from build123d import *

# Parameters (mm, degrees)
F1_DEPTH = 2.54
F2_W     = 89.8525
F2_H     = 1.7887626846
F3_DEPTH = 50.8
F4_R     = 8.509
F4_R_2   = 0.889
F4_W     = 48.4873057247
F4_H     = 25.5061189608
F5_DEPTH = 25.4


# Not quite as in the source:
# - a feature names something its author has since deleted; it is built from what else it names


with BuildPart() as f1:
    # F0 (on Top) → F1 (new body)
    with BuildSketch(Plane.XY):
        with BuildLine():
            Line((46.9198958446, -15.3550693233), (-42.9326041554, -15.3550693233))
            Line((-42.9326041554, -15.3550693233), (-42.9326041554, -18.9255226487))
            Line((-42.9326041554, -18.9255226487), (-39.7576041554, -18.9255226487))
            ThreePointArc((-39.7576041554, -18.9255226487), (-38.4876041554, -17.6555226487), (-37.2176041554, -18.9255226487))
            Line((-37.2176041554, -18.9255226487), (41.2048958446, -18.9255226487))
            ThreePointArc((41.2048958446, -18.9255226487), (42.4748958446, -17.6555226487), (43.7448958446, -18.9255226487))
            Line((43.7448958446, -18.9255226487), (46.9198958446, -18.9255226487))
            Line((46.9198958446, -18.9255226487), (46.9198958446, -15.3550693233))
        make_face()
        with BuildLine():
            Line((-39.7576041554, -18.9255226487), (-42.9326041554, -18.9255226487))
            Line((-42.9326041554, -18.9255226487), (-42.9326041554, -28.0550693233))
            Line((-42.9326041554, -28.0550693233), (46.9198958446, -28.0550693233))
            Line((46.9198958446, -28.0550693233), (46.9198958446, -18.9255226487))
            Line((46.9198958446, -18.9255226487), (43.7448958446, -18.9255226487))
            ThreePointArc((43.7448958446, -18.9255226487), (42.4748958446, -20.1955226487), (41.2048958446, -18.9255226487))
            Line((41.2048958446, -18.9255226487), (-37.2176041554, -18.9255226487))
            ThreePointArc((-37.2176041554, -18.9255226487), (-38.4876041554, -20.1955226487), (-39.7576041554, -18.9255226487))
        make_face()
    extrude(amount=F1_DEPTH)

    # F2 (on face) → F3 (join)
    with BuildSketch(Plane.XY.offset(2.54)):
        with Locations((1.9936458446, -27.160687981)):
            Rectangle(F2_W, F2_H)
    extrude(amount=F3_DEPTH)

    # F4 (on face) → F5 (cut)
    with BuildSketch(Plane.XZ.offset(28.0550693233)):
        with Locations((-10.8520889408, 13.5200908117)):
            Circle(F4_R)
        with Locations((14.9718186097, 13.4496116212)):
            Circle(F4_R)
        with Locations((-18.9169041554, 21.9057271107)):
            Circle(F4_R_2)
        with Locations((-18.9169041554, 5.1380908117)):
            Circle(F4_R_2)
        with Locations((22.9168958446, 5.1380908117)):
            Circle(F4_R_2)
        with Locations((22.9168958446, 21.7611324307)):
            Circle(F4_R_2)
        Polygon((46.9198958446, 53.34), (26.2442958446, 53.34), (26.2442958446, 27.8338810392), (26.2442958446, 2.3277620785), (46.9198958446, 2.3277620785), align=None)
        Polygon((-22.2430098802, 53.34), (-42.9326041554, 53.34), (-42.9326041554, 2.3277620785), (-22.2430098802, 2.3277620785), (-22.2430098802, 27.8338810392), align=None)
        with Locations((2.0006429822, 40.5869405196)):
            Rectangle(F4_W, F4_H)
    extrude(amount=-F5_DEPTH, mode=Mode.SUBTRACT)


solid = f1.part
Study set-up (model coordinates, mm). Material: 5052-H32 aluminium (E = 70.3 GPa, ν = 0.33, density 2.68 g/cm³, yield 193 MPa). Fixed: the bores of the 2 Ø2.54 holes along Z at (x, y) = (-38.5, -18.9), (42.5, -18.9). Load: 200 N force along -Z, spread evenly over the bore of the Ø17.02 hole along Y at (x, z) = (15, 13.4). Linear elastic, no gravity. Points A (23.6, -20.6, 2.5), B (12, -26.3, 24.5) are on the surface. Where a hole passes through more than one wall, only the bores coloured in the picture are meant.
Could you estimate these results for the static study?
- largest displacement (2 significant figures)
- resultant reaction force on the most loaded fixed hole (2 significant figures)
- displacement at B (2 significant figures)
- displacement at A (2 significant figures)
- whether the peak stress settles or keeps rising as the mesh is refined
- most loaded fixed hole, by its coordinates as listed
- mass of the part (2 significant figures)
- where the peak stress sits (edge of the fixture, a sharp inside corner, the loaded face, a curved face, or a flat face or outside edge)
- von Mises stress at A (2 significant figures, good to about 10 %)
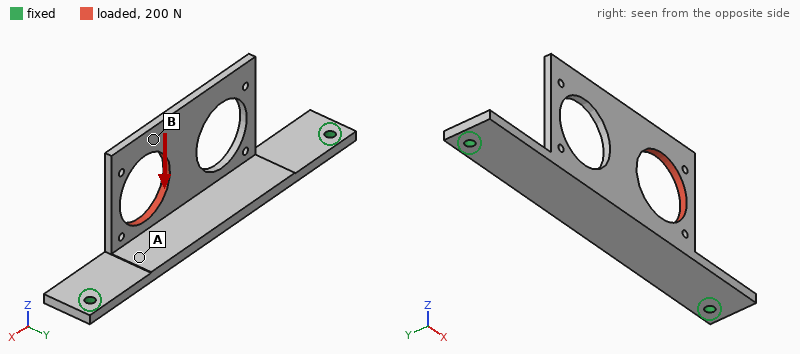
0.31 mm
150 N
0.25 mm
0.11 mm
keeps rising
(42.5, -18.9)
11 g
edge of the fixture
44 MPa
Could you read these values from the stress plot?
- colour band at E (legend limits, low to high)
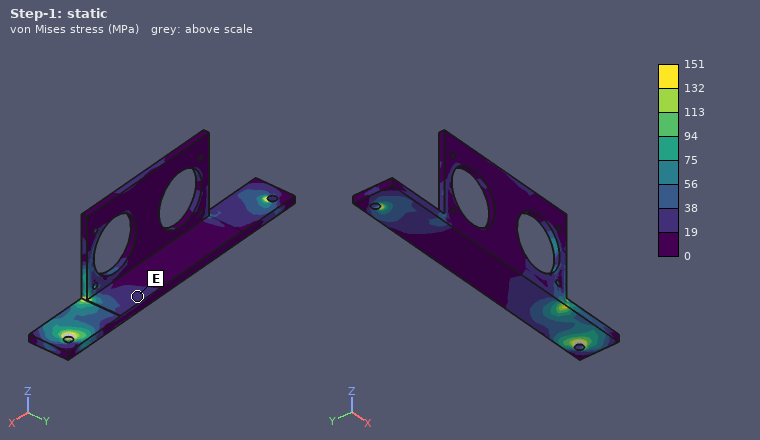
19 to 38 MPa
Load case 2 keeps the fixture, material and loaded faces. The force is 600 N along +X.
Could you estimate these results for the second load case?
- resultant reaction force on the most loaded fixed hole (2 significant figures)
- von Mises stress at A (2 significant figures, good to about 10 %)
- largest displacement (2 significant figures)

330 N
53 MPa
0.19 mm
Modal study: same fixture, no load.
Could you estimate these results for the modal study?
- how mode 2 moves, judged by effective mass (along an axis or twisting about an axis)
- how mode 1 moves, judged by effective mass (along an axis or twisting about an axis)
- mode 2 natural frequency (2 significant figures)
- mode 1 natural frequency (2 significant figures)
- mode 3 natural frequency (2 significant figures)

along Z
along Y
2300 Hz
1100 Hz
2600 Hz
